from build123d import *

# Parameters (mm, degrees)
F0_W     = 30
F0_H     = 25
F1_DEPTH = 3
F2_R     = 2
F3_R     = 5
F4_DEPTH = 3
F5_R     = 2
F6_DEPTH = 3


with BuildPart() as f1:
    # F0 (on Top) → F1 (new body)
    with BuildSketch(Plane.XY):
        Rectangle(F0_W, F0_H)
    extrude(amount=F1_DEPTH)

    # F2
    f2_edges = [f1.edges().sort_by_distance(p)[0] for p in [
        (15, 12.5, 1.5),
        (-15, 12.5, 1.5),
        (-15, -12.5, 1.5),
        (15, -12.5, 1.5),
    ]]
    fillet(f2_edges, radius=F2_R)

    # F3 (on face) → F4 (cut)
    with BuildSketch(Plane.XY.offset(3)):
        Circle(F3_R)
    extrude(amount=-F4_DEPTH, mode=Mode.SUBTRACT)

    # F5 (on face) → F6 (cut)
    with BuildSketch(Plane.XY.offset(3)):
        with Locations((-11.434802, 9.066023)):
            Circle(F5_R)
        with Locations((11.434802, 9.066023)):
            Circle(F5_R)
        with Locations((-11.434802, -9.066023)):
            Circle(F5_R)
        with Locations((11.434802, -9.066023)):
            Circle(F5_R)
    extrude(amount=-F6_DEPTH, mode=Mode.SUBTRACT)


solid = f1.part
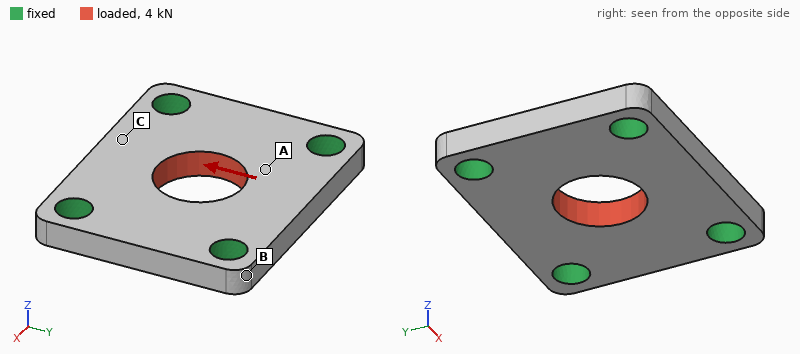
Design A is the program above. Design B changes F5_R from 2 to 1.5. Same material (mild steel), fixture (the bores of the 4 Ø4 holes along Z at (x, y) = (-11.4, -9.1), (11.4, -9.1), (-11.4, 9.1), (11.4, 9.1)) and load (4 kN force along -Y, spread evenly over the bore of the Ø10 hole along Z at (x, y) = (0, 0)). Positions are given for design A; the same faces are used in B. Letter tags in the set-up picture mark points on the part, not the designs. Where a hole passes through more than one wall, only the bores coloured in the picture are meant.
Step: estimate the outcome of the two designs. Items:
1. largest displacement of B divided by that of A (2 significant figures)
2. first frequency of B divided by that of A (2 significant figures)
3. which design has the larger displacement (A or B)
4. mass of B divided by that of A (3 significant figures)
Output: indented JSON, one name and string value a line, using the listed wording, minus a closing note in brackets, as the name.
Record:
{
  "largest displacement of B divided by that of A": "1.1",
  "first frequency of B divided by that of A": "0.88",
  "which design has the larger displacement": "B",
  "mass of B divided by that of A": "1.04"
}
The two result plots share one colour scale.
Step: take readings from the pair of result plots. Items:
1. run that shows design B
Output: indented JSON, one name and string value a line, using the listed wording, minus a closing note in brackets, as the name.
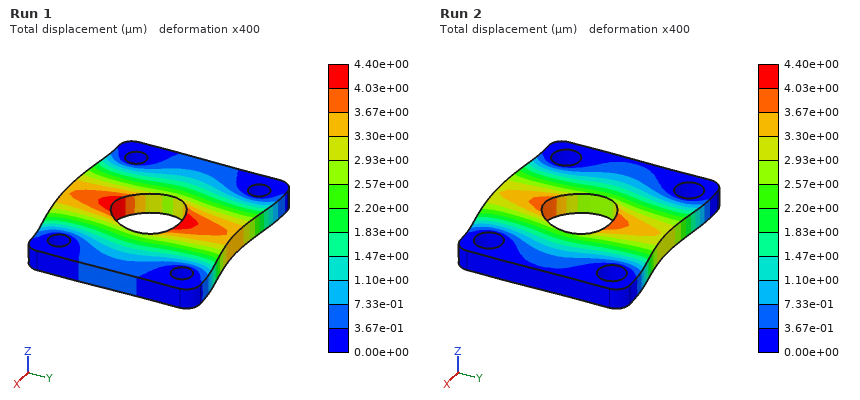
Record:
{
  "run that shows design B": "Run 1"
}
